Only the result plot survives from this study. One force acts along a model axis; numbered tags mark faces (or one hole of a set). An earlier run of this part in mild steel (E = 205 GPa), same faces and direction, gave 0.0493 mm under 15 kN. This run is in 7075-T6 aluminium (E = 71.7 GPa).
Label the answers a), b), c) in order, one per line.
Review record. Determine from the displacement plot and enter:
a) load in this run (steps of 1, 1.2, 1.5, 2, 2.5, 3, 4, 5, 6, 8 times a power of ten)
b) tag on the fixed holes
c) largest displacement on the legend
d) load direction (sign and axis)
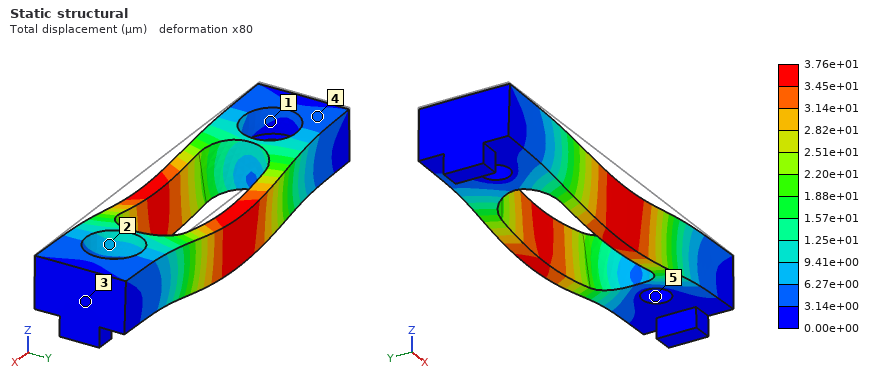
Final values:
a) 4 kN
b) 5
c) 3.76e+01 µm
d) -Z
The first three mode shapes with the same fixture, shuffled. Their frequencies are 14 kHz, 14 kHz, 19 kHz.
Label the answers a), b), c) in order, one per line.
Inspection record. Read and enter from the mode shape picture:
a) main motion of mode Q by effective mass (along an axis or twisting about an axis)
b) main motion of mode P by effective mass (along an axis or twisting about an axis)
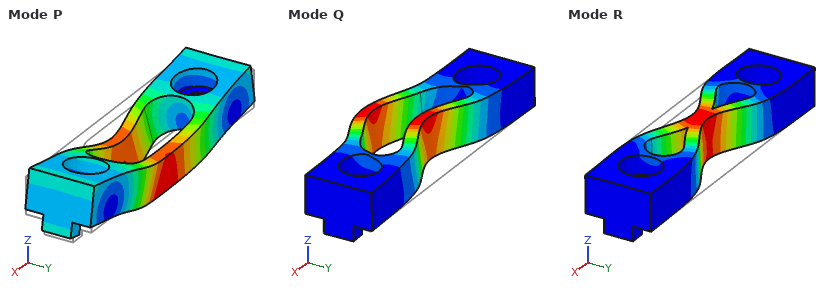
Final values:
a) along Y
b) along Z
